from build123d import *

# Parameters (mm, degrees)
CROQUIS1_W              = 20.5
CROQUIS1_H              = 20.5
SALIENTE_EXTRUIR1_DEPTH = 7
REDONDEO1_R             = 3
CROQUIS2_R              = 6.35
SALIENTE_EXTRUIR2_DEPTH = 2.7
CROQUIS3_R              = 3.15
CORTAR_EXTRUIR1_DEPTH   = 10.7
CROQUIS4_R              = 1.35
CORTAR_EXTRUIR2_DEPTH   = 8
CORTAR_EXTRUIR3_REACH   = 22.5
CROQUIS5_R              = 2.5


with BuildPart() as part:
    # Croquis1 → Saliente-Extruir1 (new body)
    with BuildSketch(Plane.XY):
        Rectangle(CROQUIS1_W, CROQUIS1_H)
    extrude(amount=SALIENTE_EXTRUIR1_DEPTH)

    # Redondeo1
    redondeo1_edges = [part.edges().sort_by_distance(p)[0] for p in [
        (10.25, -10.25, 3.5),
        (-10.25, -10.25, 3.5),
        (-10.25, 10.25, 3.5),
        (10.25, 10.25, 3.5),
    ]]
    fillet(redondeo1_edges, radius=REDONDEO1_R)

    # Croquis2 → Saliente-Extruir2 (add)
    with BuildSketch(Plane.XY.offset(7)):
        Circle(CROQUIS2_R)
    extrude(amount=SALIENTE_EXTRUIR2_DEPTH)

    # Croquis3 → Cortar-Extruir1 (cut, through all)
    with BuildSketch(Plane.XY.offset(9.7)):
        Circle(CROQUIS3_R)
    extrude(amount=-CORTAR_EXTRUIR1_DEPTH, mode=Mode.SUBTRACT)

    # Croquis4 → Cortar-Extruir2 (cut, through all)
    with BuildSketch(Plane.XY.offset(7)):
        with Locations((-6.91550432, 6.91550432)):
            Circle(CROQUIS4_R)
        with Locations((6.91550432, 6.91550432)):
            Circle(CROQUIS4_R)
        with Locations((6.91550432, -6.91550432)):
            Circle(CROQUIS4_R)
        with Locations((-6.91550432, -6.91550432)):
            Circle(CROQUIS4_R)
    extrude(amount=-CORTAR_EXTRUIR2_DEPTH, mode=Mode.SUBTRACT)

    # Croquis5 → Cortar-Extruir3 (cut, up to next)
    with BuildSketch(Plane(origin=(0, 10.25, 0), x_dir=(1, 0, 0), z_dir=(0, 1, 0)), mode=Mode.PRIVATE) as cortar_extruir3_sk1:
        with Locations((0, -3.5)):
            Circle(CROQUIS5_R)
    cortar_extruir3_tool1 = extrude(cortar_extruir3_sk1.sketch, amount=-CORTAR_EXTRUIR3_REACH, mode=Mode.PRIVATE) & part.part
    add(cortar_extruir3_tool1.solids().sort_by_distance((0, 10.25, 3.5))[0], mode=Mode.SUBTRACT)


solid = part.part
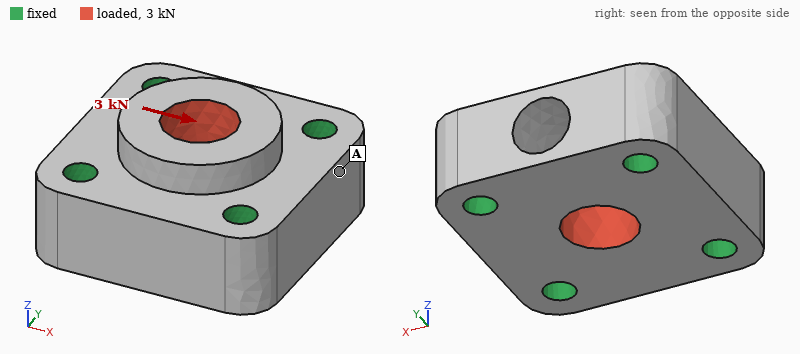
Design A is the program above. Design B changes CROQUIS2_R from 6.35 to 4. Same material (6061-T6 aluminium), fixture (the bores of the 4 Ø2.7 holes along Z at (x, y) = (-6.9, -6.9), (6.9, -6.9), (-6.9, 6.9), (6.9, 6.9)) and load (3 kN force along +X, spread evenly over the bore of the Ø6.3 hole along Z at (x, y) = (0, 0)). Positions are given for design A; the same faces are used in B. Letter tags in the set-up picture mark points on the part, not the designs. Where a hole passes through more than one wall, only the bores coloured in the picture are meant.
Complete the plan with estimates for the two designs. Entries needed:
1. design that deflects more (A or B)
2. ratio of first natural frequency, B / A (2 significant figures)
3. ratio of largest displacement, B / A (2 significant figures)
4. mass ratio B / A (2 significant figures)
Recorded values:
B
1.0
2.9
0.92
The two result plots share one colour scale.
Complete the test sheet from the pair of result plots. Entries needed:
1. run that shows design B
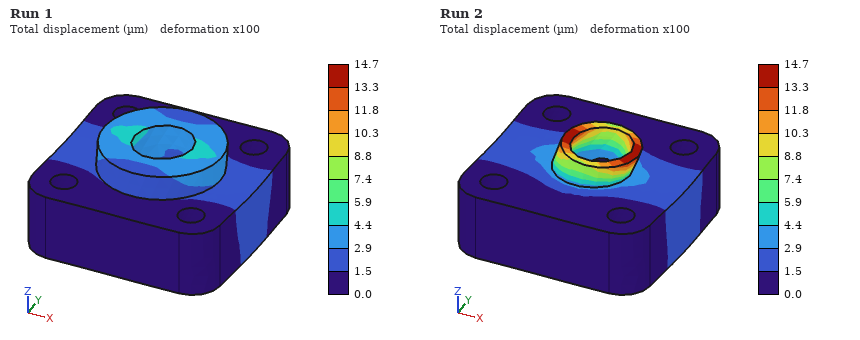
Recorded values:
Run 2
